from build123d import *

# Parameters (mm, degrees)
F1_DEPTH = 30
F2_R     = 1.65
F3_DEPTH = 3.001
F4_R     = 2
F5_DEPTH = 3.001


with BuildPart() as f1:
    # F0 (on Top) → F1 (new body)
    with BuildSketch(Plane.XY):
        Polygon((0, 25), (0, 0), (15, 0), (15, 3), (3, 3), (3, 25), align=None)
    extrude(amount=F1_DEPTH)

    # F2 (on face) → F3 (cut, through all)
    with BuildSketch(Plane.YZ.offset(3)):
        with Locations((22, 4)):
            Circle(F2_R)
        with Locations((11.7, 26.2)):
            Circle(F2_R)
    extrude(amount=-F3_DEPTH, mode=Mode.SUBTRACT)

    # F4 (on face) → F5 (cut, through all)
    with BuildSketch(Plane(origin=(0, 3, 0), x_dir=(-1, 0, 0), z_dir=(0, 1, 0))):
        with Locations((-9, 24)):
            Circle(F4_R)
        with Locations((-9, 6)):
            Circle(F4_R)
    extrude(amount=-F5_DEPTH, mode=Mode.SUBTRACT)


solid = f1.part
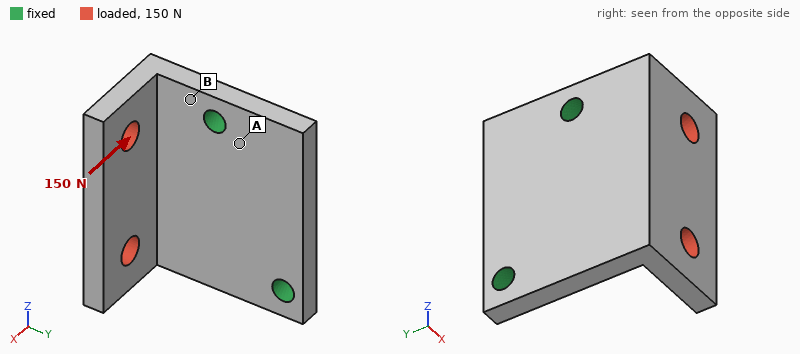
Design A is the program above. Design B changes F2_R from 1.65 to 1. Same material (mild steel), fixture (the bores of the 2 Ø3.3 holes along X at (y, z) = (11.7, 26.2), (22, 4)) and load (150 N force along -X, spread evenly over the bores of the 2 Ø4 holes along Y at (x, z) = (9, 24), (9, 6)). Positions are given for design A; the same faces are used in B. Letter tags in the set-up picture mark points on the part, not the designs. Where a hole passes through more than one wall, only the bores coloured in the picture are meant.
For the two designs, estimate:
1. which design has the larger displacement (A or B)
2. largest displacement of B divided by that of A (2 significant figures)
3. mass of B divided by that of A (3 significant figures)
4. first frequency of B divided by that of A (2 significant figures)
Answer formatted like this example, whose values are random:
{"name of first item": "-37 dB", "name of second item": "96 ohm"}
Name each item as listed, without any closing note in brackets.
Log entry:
{"which design has the larger displacement": "B", "largest displacement of B divided by that of A": "1.2", "mass of B divided by that of A": "1.01", "first frequency of B divided by that of A": "0.91"}
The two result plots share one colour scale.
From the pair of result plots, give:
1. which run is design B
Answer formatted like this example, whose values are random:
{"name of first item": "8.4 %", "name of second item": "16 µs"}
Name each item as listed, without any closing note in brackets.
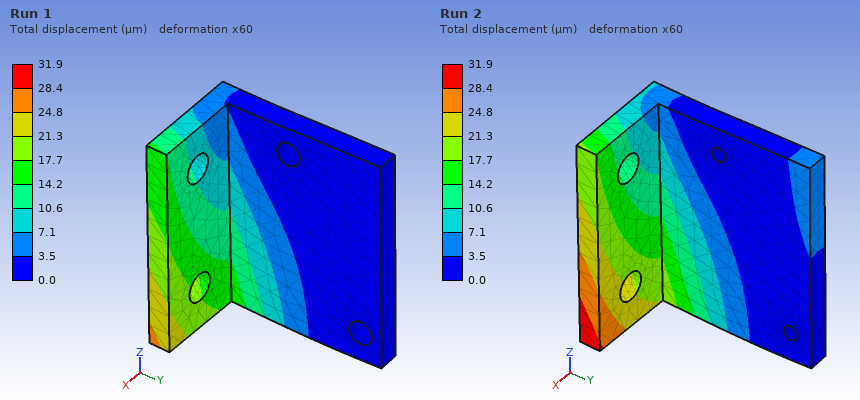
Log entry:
{"which run is design B": "Run 2"}
